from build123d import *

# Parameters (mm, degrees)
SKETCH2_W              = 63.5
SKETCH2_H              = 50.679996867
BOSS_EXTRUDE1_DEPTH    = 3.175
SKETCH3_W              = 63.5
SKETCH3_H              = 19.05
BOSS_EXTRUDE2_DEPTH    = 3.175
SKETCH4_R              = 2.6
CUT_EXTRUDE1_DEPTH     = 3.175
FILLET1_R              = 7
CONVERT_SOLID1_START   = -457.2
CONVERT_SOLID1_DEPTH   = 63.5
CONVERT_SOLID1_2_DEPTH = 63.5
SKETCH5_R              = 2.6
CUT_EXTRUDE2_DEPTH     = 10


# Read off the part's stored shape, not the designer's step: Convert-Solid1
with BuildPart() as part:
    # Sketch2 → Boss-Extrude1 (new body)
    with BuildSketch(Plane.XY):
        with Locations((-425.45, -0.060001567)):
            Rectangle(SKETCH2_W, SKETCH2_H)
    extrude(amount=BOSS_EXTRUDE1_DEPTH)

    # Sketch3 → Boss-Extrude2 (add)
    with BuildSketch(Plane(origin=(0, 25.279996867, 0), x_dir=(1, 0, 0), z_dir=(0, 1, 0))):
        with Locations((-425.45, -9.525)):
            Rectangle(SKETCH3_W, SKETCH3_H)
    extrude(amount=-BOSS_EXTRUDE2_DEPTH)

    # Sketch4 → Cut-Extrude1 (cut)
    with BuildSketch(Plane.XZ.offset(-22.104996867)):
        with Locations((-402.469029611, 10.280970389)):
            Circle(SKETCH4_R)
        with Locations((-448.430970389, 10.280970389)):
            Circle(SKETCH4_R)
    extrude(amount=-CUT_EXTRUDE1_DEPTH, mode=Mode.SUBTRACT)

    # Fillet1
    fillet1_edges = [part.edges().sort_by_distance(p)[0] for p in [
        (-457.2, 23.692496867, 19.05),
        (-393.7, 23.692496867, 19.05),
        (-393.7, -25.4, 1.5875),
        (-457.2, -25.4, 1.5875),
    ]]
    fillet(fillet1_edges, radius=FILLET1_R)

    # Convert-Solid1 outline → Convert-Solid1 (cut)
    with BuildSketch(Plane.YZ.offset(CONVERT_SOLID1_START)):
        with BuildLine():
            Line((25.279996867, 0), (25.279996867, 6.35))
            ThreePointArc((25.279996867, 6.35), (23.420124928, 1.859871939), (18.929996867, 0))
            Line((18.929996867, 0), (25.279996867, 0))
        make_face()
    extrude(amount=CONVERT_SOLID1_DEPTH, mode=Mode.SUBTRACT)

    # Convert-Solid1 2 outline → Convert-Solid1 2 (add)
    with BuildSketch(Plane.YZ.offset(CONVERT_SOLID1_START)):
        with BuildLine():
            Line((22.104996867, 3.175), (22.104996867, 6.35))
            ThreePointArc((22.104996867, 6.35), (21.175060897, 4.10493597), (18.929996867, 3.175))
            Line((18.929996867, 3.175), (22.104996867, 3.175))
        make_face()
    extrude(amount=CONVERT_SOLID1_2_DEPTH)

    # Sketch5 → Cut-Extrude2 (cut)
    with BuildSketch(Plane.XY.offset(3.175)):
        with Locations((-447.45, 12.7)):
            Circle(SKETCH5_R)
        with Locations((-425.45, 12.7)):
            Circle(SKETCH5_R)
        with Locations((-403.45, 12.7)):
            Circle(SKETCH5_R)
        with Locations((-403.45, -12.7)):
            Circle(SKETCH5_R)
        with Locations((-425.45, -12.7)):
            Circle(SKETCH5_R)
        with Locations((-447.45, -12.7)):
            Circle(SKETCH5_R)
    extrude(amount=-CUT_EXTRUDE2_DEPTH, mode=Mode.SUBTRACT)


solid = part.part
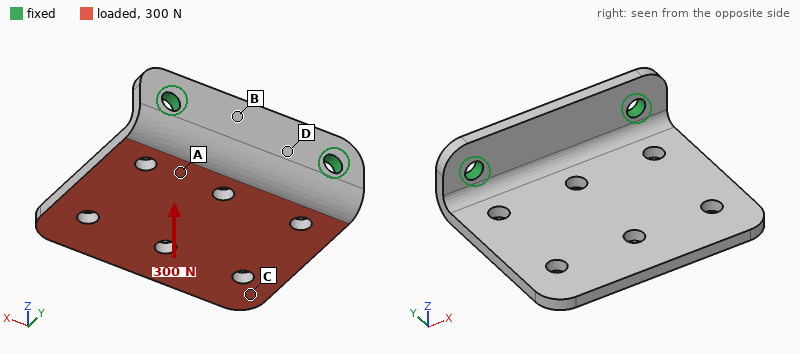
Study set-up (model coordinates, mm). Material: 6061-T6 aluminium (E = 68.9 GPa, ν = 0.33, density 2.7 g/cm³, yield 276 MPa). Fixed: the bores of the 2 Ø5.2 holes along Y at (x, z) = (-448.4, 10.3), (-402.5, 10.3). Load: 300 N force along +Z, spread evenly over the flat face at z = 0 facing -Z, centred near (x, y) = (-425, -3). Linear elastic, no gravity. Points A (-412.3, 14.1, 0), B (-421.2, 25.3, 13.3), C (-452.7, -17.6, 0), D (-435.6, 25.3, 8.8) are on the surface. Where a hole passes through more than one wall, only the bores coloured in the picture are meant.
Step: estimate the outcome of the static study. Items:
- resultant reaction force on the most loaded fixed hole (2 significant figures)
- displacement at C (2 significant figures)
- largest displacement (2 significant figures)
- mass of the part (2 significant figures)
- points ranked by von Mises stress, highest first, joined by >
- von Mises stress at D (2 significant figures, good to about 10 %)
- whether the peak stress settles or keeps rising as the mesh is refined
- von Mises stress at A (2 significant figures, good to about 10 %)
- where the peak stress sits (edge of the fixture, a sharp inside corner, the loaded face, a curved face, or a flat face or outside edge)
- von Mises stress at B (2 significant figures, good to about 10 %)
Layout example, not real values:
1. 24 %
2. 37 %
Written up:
1. 150 N
2. 0.55 mm
3. 0.69 mm
4. 33 g
5. A > D > B > C
6. 39 MPa
7. keeps rising
8. 52 MPa
9. edge of the fixture
10. 24 MPa
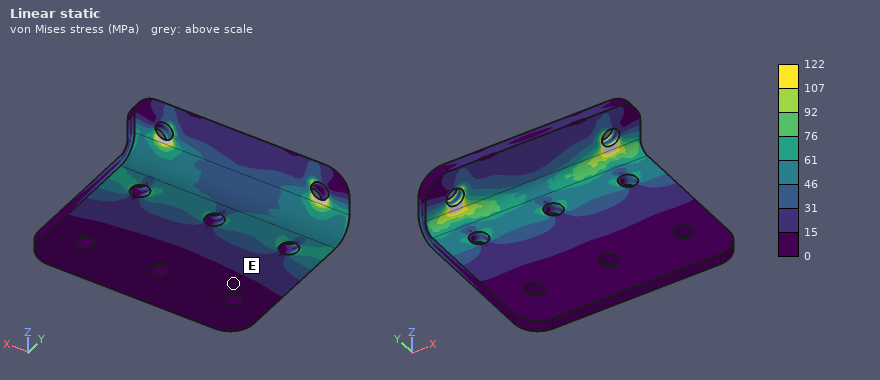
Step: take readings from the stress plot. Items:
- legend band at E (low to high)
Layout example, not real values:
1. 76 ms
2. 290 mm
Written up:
1. 0 to 15 MPa
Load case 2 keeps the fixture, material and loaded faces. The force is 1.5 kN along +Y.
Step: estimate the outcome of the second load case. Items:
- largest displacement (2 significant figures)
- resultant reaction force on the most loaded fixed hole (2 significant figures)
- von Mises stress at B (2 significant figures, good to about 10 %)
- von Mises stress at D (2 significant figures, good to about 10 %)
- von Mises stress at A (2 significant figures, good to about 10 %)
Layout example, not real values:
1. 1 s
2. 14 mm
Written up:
1. 0.52 mm
2. 760 N
3. 17 MPa
4. 35 MPa
5. 28 MPa
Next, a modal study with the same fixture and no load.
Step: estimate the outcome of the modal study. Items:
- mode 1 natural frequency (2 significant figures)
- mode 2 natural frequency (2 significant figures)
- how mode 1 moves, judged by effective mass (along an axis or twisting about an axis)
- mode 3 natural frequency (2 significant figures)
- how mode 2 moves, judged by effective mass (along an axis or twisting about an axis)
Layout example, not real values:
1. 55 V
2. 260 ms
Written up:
1. 860 Hz
2. 2000 Hz
3. along Z
4. 5000 Hz
5. twisting about Y
